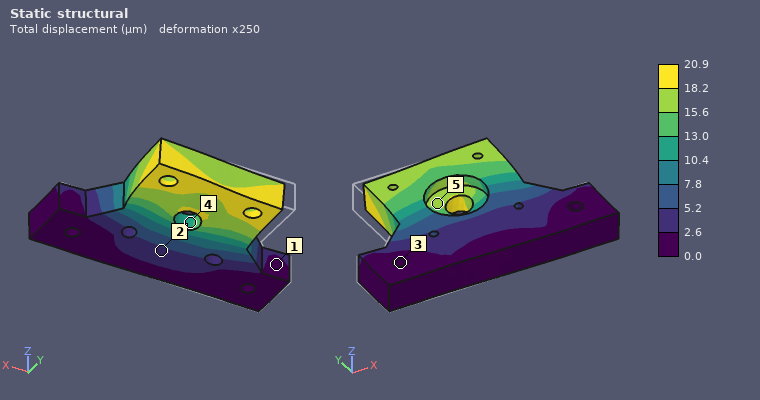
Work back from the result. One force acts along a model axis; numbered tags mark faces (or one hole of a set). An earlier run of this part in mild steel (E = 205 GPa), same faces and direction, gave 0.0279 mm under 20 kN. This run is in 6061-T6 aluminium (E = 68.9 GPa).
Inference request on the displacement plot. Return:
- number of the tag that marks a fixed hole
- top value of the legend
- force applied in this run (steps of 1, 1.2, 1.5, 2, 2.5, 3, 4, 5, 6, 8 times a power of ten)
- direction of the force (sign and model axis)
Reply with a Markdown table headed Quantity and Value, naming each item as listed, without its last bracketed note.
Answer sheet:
| Quantity | Value |
|---|---|
| number of the tag that marks a fixed hole | 3 |
| top value of the legend | 20.9 µm |
| force applied in this run | 5 kN |
| direction of the force | +X |
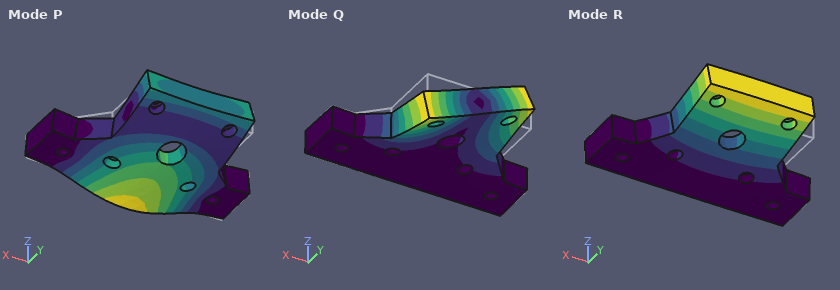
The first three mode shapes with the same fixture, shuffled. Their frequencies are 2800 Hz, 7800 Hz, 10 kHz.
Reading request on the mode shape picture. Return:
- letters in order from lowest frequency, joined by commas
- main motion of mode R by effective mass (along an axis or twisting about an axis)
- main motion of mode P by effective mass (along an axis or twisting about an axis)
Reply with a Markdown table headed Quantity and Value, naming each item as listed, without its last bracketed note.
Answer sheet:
| Quantity | Value |
|---|---|
| letters in order from lowest frequency, joined by commas | R, Q, P |
| main motion of mode R by effective mass | along Z |
| main motion of mode P by effective mass | along Z |
